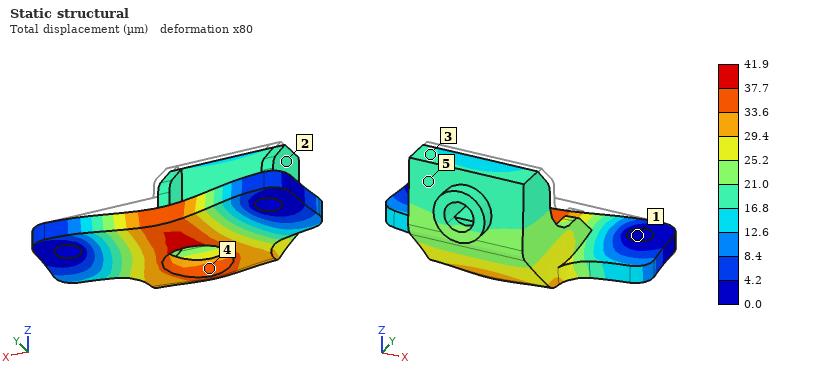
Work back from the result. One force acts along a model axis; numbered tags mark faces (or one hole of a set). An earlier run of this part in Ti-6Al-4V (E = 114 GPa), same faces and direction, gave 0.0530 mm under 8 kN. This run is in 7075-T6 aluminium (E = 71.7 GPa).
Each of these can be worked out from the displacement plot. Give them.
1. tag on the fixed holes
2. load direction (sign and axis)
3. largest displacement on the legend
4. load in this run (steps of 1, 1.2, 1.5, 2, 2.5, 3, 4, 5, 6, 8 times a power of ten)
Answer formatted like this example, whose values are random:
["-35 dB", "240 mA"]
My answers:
["1", "-Y", "41.9 µm", "4 kN"]
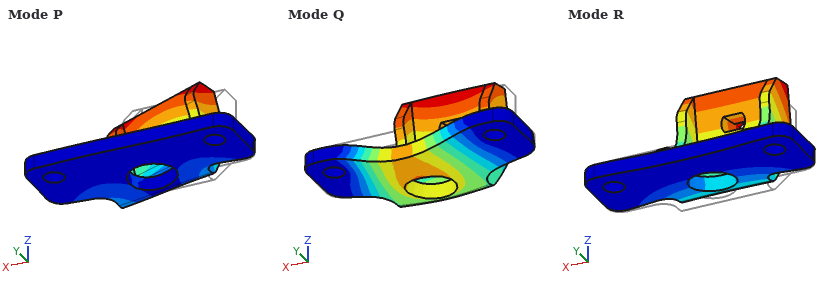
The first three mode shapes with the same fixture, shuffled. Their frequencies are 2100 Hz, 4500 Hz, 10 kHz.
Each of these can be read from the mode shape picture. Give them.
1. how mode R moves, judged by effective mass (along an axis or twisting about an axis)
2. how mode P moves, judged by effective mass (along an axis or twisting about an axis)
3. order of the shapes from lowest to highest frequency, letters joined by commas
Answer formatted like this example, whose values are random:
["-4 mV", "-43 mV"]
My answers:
["along Z", "along X", "R, P, Q"]
